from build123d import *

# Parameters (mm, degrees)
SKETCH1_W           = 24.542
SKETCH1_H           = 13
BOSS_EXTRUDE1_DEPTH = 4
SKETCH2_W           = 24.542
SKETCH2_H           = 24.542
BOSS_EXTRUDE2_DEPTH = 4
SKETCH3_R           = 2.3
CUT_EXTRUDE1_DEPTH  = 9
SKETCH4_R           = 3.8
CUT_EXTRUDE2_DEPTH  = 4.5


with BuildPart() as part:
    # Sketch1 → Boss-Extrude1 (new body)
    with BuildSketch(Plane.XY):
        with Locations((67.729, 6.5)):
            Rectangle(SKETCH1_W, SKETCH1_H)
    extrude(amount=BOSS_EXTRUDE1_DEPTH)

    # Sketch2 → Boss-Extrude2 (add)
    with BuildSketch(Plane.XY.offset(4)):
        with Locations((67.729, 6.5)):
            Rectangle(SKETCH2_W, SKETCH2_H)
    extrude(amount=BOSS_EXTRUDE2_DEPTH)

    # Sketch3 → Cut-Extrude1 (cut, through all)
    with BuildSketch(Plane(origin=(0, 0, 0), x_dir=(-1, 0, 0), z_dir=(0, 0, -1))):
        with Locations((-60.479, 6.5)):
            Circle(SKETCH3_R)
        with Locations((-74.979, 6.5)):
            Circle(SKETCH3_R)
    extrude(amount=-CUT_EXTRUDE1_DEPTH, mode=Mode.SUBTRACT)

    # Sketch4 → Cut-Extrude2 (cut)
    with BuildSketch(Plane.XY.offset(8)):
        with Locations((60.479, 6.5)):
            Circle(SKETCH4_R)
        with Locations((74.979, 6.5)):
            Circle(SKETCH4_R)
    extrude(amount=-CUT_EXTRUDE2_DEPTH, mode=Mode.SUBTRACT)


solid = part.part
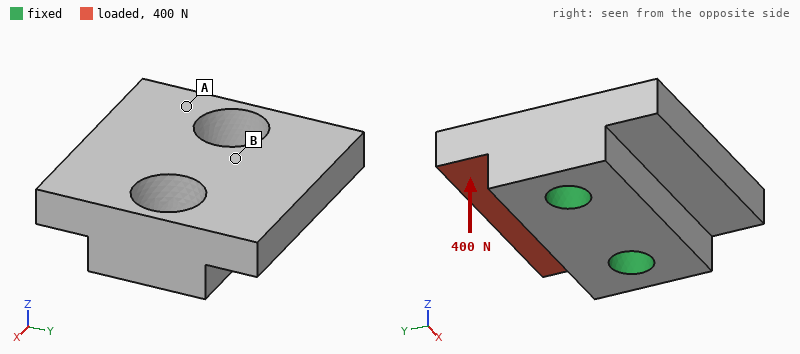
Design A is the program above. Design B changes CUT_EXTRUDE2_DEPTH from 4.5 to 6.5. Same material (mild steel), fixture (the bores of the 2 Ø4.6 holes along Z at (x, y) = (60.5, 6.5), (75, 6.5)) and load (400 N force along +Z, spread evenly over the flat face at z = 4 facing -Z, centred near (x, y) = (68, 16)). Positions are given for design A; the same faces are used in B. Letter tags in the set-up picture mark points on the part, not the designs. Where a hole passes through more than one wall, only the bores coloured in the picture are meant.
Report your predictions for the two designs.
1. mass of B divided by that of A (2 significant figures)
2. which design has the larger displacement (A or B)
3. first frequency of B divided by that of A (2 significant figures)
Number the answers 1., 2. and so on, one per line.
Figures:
1. 0.96
2. B
3. 0.51
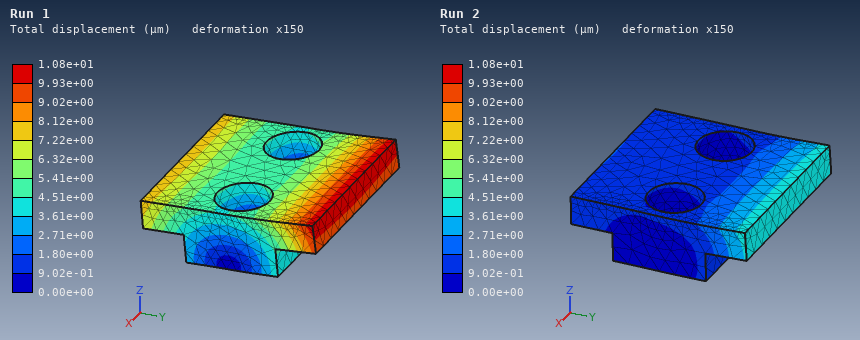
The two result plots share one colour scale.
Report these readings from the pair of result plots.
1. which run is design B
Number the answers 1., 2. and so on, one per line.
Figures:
1. Run 1
